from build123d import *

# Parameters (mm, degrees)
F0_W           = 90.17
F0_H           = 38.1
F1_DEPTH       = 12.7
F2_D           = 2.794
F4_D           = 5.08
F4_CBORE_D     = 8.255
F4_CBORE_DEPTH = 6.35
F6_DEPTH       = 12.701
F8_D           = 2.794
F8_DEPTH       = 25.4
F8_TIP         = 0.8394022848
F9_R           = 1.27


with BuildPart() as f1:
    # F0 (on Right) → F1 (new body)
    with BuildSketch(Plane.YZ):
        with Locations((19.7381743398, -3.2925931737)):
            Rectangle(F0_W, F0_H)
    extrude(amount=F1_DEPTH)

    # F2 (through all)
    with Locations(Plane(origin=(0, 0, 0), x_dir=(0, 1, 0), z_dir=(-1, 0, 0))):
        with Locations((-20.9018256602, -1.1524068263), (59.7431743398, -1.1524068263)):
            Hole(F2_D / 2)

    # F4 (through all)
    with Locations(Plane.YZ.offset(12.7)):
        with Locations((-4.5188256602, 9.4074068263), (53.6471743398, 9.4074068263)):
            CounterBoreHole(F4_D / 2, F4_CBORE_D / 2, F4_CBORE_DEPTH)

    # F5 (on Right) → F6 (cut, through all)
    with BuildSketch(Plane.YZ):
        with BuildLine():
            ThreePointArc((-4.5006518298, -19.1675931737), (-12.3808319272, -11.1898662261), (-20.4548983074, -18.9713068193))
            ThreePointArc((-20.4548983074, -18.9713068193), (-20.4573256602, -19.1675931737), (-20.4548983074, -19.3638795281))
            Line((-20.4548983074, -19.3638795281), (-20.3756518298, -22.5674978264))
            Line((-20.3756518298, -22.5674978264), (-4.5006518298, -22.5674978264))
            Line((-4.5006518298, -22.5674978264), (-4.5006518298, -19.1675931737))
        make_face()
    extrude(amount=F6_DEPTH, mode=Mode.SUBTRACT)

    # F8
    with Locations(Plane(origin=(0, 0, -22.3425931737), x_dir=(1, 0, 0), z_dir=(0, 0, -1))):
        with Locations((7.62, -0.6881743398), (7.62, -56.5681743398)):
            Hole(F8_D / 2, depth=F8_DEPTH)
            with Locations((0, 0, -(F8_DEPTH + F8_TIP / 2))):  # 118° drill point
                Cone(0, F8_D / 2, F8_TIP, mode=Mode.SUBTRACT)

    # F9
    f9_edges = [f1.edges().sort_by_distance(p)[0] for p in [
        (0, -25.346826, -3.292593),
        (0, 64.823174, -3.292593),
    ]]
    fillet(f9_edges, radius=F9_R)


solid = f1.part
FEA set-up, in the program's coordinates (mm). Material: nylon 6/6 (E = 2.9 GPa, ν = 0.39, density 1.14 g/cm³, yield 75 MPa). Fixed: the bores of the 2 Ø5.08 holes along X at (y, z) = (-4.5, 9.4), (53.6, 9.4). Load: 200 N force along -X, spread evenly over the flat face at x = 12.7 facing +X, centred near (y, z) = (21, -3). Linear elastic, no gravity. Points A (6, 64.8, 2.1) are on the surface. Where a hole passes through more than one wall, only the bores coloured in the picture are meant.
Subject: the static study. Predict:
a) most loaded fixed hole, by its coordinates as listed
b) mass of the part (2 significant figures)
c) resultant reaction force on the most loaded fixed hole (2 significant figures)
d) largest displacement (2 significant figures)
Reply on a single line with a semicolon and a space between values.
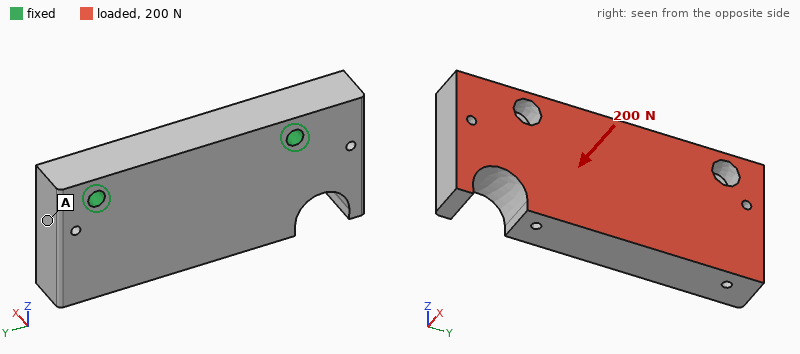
(-4.5, 9.4); 46 g; 110 N; 0.11 mm
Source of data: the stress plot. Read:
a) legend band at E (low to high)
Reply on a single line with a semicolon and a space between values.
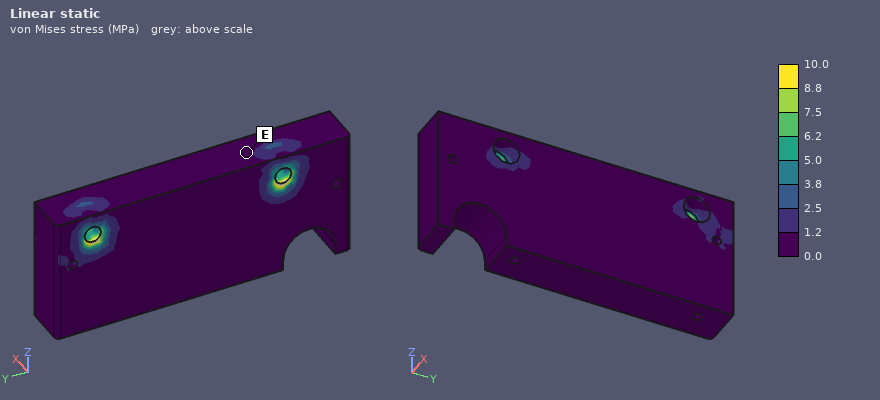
0.0 to 1.2 MPa
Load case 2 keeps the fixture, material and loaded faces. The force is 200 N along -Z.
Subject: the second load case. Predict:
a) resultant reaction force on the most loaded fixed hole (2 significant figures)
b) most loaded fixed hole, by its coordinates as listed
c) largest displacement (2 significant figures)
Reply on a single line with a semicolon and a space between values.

110 N; (-4.5, 9.4); 79 µm
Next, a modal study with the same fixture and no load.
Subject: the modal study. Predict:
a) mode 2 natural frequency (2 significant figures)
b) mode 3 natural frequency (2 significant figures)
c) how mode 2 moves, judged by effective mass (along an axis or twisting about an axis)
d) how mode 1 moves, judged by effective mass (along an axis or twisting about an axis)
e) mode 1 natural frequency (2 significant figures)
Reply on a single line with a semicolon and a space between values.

2400 Hz; 3200 Hz; twisting about Z; along X; 1200 Hz
